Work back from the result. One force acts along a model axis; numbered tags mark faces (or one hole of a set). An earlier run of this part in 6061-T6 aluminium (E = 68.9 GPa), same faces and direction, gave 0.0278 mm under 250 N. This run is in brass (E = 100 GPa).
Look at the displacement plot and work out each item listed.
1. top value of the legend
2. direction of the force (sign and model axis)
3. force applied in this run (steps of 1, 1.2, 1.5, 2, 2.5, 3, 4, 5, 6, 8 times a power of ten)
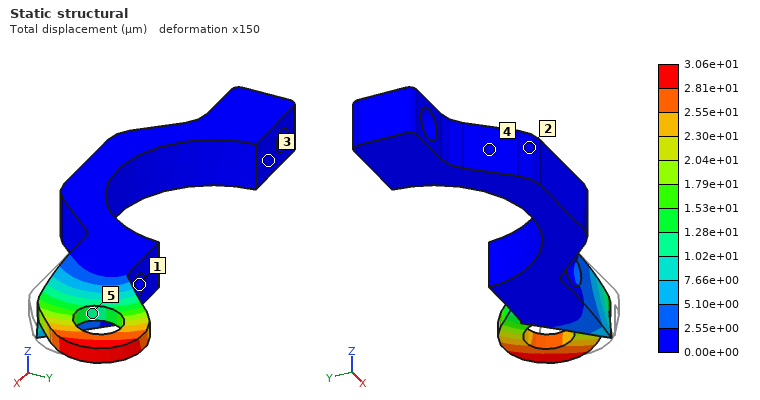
3.06e+01 µm
+Y
400 N
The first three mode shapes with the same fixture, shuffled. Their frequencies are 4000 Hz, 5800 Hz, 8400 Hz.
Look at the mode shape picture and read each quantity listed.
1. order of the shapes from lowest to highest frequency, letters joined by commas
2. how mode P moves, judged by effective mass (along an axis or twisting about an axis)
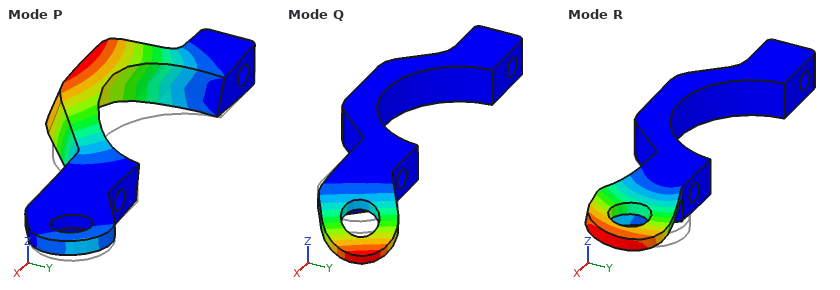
Q, P, R
along Z
